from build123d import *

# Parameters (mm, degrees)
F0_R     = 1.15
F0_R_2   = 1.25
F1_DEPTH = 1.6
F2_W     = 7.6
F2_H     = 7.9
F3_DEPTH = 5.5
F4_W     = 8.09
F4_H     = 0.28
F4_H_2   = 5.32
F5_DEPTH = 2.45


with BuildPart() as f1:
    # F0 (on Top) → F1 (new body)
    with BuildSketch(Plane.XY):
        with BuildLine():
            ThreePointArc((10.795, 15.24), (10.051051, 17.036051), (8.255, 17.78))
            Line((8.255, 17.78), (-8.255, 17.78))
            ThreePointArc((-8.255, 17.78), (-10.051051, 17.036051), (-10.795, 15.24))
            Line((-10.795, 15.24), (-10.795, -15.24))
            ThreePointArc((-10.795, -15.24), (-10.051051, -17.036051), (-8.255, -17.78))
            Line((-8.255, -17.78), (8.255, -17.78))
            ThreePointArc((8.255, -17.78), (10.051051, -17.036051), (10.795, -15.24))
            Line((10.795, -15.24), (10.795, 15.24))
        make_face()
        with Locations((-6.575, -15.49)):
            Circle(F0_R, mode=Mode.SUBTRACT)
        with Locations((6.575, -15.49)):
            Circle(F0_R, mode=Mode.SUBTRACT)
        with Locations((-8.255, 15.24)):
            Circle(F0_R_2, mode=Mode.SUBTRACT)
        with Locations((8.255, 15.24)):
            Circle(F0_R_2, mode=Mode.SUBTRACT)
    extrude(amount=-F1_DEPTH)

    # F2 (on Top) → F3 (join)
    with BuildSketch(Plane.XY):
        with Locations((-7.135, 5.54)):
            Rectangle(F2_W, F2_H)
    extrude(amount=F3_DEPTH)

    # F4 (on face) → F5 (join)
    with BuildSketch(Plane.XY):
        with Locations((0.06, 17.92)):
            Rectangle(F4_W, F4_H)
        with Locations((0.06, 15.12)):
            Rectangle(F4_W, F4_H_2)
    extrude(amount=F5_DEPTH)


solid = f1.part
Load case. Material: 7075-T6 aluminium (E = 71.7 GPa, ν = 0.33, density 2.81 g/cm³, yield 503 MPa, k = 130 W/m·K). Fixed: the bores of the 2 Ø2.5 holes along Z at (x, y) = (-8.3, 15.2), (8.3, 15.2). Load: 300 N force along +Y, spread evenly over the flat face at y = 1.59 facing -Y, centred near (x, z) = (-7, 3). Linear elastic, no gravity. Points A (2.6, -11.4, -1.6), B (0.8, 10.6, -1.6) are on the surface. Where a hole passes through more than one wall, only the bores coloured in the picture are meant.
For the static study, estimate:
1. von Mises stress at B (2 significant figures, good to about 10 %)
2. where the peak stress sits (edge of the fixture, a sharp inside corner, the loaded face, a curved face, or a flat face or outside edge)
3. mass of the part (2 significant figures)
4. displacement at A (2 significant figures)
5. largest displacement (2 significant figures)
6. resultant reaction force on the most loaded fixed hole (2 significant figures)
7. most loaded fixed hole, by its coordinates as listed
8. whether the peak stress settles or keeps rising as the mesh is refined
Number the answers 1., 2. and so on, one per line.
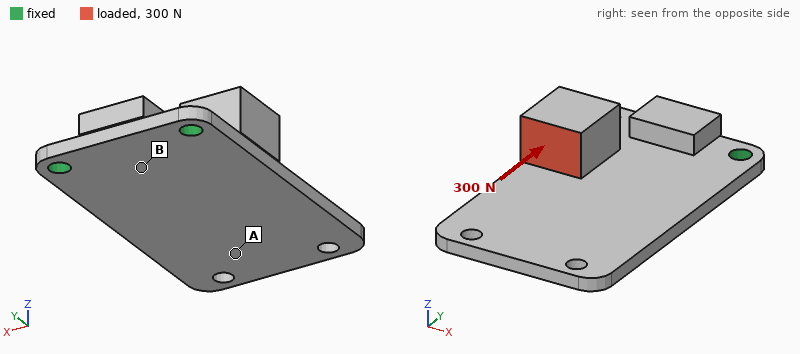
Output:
1. 87 MPa
2. edge of the fixture
3. 4.6 g
4. 0.32 mm
5. 0.46 mm
6. 280 N
7. (-8.3, 15.2)
8. keeps rising
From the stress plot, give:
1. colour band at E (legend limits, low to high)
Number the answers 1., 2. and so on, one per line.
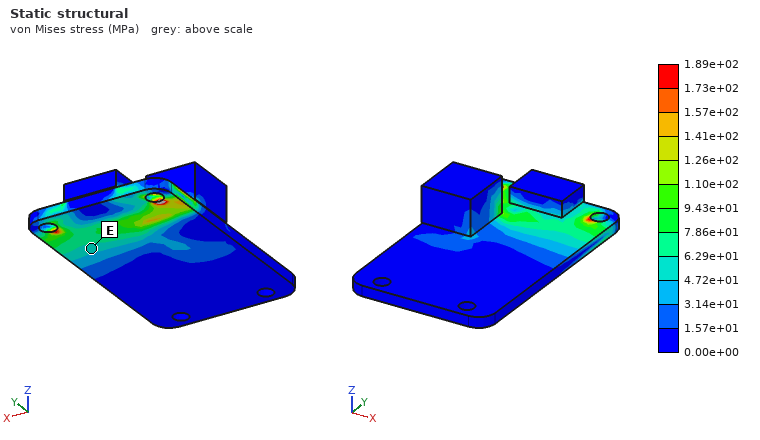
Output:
1. 4.72e+01 to 6.29e+01 MPa
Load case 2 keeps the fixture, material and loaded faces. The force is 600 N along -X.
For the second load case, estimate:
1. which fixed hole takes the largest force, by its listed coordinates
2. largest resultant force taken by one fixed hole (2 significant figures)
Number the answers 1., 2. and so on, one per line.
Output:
1. (8.3, 15.2)
2. 610 N
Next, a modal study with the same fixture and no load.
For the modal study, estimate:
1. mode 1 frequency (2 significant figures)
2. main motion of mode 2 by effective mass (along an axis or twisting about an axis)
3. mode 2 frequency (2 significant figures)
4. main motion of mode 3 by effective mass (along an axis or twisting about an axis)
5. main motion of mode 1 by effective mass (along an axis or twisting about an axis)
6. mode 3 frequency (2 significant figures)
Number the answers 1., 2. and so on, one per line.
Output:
1. 1300 Hz
2. twisting about Y
3. 4700 Hz
4. along Z
5. along Z
6. 7000 Hz
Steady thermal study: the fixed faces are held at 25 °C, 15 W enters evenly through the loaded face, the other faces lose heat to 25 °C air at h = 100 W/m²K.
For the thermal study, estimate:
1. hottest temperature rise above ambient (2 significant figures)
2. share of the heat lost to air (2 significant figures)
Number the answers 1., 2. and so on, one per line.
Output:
1. 44 K
2. 25 %
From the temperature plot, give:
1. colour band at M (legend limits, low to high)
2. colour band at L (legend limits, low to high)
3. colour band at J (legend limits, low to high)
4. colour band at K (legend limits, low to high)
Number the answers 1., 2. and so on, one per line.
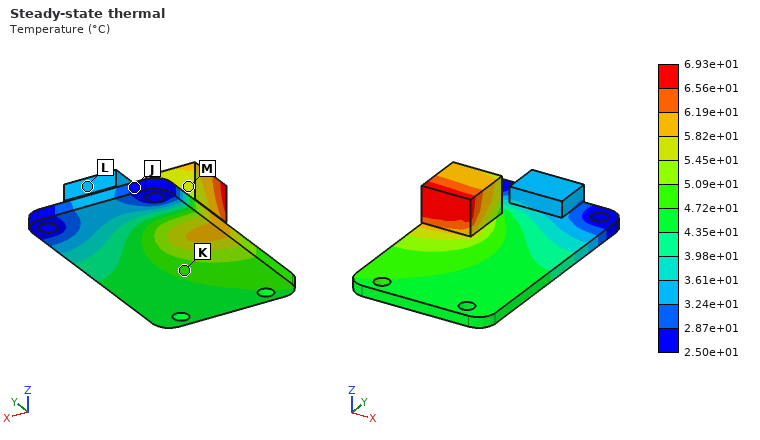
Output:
1. 5.45e+01 to 5.82e+01 °C
2. 3.24e+01 to 3.61e+01 °C
3. 2.50e+01 to 2.87e+01 °C
4. 4.72e+01 to 5.09e+01 °C
